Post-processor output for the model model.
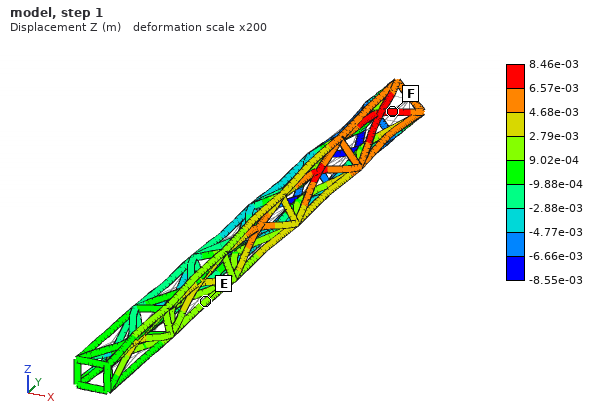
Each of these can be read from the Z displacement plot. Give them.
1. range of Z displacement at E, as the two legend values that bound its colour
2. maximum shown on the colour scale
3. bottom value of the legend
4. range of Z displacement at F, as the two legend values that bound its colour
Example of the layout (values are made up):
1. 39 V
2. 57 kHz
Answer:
1. 9.02e-04 to 2.79e-03 m
2. 8.46e-03 m
3. -8.55e-03 m
4. 6.57e-03 to 8.46e-03 m
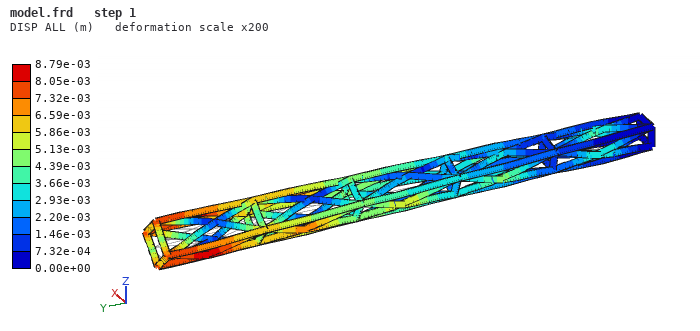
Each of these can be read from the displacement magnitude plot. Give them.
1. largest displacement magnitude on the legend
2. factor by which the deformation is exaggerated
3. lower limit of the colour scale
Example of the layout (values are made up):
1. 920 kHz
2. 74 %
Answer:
1. 8.79e-03 m
2. 200
3. 0.00e+00 m
